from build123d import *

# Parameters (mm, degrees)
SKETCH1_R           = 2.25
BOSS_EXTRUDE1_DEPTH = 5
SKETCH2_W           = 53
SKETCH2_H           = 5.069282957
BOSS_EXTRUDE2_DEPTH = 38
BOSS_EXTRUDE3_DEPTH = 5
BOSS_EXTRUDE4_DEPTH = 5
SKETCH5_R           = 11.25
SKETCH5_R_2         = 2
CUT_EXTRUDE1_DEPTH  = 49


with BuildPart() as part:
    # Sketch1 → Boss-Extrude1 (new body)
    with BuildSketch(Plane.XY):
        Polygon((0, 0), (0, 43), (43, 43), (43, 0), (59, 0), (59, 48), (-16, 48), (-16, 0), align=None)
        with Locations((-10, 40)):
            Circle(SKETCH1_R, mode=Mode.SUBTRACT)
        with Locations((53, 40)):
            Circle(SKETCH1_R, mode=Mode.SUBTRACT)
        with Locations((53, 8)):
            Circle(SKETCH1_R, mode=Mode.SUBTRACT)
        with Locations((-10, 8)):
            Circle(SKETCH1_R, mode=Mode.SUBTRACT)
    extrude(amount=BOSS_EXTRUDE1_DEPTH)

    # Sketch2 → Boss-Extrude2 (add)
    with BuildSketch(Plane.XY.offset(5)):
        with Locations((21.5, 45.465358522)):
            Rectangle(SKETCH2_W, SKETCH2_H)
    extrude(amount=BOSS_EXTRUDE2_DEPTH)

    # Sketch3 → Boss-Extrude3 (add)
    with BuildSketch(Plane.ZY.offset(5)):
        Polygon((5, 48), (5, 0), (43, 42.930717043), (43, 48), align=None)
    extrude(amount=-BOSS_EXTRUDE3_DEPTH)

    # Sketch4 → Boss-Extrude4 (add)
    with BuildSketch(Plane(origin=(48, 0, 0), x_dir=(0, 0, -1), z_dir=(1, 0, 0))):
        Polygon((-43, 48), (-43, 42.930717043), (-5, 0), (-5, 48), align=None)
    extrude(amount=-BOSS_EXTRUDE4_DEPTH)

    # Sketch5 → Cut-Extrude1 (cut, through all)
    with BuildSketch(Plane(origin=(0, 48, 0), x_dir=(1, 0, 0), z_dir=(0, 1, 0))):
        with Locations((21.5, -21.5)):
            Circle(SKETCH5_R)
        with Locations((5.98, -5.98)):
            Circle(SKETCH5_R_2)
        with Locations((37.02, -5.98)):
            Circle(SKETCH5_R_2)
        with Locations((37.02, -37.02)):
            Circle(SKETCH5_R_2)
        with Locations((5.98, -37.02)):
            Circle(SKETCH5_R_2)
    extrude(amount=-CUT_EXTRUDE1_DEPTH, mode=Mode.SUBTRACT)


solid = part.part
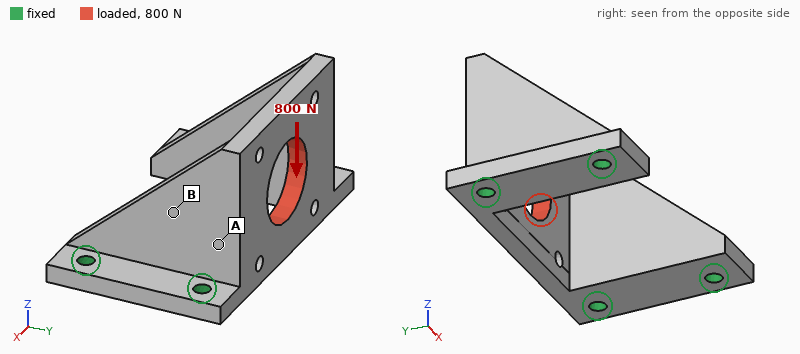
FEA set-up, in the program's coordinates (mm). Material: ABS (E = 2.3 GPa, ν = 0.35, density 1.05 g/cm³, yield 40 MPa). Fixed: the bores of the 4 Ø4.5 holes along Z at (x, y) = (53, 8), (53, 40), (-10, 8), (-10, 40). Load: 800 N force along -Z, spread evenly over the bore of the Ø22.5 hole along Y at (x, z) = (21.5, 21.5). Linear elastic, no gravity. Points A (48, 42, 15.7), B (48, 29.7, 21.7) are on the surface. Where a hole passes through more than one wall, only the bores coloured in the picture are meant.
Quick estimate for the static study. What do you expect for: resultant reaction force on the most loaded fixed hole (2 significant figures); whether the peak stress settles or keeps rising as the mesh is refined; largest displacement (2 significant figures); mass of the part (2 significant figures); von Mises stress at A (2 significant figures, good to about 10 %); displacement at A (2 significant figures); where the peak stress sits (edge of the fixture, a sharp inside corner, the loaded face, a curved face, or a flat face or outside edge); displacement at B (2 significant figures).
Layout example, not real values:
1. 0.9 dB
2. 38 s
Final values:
1. 490 N
2. keeps rising
3. 0.34 mm
4. 26 g
5. 5.5 MPa
6. 0.14 mm
7. edge of the fixture
8. 0.12 mm
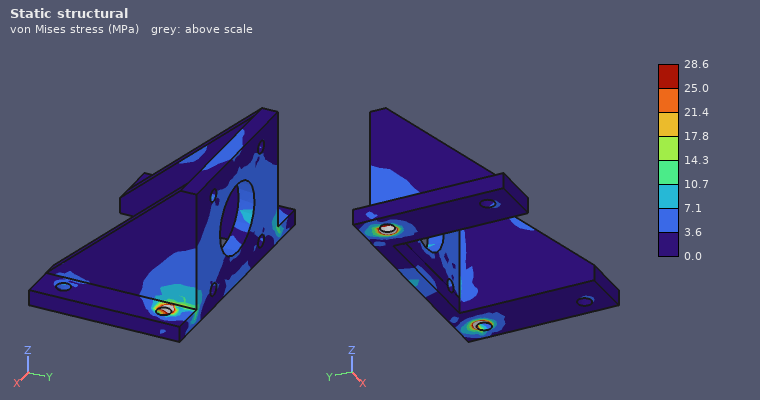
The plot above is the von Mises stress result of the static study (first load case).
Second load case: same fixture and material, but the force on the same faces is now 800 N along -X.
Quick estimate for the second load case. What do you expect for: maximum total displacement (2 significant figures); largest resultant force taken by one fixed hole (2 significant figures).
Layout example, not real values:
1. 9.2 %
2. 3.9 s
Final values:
1. 0.33 mm
2. 510 N
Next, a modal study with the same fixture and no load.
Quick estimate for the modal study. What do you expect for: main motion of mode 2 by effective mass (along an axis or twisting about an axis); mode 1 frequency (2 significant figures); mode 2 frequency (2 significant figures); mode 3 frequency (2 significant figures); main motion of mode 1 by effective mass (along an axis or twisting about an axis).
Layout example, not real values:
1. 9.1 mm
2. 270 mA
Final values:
1. along X
2. 1800 Hz
3. 2200 Hz
4. 2700 Hz
5. along Y
